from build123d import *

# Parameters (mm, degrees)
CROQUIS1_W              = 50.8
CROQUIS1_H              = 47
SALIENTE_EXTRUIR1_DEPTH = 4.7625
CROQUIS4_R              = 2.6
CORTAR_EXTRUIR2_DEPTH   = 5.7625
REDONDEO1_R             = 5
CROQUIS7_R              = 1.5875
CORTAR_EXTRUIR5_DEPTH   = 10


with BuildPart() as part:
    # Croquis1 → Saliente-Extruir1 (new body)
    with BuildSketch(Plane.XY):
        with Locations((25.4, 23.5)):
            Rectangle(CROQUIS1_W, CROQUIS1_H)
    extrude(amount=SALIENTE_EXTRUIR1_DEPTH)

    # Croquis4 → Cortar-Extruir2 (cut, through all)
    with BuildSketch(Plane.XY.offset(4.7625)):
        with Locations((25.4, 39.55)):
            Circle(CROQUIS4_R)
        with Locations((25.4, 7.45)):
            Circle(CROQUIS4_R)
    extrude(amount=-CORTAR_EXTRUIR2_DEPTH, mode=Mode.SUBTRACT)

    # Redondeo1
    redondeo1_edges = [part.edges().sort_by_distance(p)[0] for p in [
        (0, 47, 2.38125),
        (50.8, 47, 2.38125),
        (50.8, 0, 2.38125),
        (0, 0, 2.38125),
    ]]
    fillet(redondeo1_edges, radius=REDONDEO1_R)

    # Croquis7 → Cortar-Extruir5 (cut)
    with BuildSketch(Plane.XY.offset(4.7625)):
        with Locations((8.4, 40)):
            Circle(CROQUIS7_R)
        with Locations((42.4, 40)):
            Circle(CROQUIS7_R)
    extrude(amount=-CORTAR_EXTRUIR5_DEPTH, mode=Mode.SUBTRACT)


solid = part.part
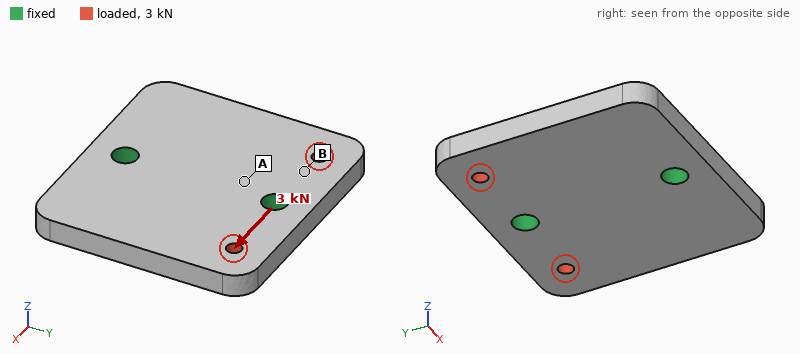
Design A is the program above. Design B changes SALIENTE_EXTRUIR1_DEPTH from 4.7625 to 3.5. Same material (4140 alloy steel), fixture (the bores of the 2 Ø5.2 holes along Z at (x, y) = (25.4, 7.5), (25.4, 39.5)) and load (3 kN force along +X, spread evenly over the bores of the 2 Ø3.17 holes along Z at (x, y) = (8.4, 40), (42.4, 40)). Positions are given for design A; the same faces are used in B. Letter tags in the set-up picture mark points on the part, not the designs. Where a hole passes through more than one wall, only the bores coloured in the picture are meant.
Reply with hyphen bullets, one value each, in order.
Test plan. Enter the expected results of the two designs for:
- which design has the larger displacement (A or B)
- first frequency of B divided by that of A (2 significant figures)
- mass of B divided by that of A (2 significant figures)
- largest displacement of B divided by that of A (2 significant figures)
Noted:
- B
- 0.77
- 0.73
- 1.4
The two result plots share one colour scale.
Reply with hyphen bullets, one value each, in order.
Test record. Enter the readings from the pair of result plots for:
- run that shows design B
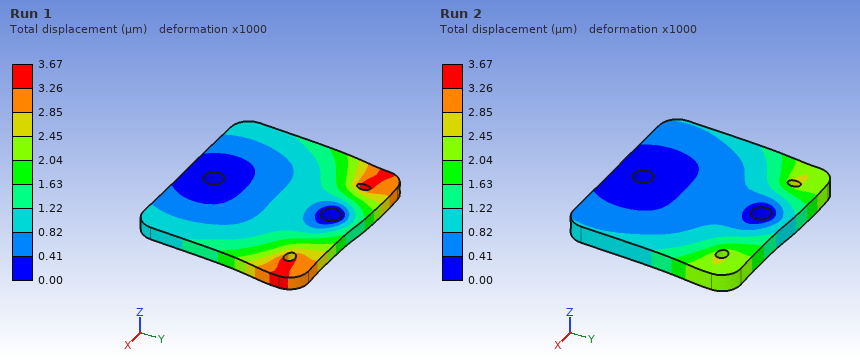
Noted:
- Run 1
